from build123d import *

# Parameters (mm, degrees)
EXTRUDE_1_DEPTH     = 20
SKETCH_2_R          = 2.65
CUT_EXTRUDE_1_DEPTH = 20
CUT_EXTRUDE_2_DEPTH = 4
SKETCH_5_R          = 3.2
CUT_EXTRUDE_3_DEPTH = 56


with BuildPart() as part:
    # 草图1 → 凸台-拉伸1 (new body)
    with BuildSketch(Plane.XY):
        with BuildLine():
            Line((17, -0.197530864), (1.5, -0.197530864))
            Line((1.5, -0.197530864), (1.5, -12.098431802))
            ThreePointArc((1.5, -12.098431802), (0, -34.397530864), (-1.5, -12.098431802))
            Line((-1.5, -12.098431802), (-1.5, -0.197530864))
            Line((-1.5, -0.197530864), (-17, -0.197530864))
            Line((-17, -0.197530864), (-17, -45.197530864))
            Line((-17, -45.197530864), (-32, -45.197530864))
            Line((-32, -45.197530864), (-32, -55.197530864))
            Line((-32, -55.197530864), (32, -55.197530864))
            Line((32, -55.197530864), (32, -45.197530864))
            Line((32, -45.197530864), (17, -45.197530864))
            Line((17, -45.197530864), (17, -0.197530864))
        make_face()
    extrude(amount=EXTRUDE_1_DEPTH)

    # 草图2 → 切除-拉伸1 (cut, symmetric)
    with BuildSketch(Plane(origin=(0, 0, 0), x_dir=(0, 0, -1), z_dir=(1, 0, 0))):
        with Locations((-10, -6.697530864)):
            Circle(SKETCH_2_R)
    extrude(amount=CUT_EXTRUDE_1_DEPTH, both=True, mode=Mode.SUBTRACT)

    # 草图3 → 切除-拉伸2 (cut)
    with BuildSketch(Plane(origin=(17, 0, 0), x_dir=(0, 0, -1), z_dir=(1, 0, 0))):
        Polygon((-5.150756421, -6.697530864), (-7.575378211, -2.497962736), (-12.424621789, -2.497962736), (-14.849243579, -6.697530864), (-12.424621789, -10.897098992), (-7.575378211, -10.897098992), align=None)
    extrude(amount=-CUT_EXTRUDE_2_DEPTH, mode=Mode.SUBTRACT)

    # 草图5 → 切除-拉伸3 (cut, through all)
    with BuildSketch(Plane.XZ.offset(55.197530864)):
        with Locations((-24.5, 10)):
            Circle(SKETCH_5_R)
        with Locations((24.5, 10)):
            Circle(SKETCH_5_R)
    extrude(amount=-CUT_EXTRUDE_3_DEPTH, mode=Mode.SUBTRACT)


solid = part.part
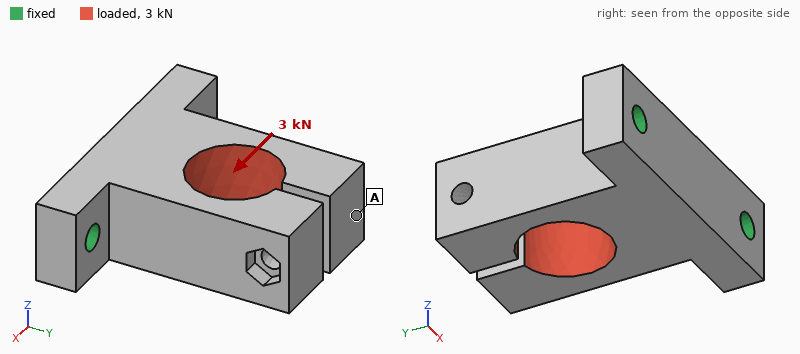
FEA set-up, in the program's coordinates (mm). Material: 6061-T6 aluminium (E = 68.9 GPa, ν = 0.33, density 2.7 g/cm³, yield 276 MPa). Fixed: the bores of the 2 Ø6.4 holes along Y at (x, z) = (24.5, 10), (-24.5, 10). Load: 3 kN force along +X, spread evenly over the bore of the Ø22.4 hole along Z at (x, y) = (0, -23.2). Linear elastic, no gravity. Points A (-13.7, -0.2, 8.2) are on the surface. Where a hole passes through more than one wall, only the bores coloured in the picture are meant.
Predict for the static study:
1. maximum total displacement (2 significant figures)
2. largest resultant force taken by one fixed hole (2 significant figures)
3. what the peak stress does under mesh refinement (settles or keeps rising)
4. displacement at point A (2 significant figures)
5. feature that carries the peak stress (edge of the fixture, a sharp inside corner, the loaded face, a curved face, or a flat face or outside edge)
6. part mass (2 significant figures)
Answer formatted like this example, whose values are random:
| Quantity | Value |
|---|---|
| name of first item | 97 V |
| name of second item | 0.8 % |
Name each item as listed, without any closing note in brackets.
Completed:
| Quantity | Value |
|---|---|
| maximum total displacement | 0.13 mm |
| largest resultant force taken by one fixed hole | 2.5 kN |
| what the peak stress does under mesh refinement | keeps rising |
| displacement at point A | 0.13 mm |
| feature that carries the peak stress | edge of the fixture |
| part mass | 90 g |
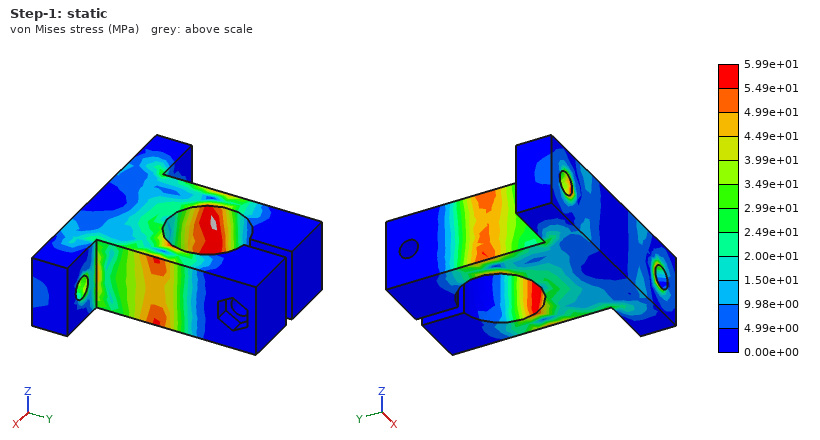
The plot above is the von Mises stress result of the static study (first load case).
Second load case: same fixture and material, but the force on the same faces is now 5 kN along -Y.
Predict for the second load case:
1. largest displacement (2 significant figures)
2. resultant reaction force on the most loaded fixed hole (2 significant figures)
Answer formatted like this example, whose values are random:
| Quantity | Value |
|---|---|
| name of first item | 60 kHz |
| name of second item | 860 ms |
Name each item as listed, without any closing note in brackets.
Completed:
| Quantity | Value |
|---|---|
| largest displacement | 0.13 mm |
| resultant reaction force on the most loaded fixed hole | 2.7 kN |
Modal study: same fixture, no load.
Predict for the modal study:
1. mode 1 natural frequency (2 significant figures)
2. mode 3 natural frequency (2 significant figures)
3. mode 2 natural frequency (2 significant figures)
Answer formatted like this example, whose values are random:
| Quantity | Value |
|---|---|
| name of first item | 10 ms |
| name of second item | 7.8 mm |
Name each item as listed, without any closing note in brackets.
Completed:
| Quantity | Value |
|---|---|
| mode 1 natural frequency | 3000 Hz |
| mode 3 natural frequency | 3100 Hz |
| mode 2 natural frequency | 3100 Hz |
